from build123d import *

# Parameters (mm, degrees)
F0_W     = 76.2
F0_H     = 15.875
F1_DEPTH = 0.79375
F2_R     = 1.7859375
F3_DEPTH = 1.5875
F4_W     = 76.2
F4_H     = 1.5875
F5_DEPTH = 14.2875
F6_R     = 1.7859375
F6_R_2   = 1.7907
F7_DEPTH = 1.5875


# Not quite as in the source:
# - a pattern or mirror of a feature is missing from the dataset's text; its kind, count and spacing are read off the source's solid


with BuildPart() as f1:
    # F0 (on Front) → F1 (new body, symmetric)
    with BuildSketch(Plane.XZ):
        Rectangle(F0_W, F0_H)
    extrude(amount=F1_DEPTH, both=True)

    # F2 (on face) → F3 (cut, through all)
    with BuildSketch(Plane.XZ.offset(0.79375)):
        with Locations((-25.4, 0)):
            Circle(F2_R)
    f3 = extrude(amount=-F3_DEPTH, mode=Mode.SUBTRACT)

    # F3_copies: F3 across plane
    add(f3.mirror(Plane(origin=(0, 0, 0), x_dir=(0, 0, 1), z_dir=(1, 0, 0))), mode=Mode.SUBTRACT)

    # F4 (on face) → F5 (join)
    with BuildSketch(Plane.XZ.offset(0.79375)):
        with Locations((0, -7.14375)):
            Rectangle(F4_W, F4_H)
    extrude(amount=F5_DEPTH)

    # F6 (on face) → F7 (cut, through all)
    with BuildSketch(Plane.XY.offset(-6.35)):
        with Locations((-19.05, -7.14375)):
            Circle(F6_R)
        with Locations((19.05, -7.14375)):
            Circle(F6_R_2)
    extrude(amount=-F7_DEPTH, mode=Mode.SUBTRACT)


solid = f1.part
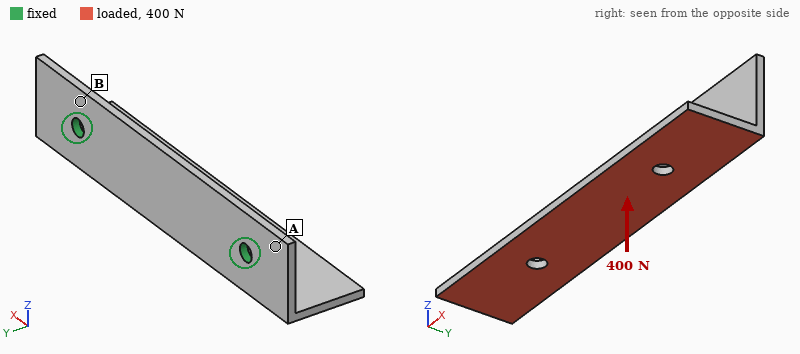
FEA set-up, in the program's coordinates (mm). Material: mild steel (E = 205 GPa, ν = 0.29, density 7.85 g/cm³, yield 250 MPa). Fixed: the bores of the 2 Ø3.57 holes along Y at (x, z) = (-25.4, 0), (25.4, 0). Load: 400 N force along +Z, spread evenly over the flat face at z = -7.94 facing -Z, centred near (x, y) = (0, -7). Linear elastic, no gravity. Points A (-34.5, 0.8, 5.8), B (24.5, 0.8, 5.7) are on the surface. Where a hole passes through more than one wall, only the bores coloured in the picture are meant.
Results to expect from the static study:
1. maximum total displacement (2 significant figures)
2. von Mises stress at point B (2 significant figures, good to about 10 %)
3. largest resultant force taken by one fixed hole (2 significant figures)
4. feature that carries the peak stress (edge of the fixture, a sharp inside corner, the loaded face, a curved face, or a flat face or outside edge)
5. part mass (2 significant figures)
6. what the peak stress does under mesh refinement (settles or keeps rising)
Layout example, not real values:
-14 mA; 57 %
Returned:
0.12 mm; 68 MPa; 200 N; edge of the fixture; 28 g; keeps rising
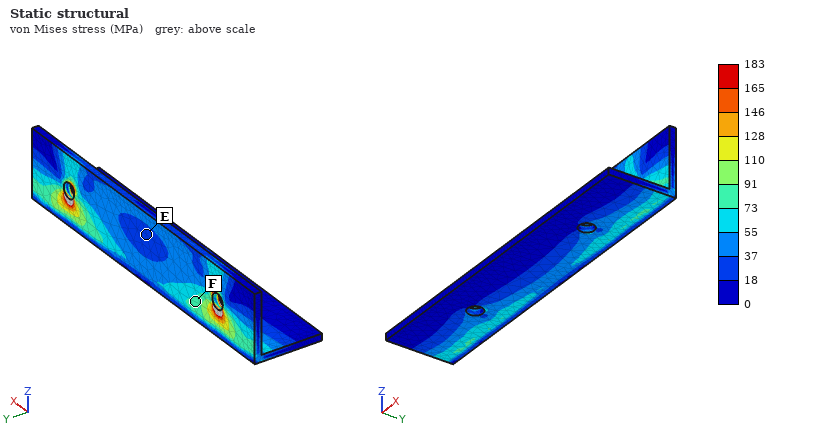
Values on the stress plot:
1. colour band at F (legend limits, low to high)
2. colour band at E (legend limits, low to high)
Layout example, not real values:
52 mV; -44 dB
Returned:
73 to 91 MPa; 18 to 37 MPa
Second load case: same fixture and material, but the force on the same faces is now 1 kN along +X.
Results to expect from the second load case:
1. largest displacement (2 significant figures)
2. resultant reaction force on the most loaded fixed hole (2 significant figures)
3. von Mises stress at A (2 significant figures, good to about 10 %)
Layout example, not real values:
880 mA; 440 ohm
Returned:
22 µm; 540 N; 14 MPa
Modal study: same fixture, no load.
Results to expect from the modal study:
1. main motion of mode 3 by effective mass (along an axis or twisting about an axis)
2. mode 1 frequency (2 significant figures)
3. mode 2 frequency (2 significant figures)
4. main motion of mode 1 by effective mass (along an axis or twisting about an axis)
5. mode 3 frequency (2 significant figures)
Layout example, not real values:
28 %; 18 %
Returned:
along Y; 2800 Hz; 3900 Hz; along Z; 5000 Hz
